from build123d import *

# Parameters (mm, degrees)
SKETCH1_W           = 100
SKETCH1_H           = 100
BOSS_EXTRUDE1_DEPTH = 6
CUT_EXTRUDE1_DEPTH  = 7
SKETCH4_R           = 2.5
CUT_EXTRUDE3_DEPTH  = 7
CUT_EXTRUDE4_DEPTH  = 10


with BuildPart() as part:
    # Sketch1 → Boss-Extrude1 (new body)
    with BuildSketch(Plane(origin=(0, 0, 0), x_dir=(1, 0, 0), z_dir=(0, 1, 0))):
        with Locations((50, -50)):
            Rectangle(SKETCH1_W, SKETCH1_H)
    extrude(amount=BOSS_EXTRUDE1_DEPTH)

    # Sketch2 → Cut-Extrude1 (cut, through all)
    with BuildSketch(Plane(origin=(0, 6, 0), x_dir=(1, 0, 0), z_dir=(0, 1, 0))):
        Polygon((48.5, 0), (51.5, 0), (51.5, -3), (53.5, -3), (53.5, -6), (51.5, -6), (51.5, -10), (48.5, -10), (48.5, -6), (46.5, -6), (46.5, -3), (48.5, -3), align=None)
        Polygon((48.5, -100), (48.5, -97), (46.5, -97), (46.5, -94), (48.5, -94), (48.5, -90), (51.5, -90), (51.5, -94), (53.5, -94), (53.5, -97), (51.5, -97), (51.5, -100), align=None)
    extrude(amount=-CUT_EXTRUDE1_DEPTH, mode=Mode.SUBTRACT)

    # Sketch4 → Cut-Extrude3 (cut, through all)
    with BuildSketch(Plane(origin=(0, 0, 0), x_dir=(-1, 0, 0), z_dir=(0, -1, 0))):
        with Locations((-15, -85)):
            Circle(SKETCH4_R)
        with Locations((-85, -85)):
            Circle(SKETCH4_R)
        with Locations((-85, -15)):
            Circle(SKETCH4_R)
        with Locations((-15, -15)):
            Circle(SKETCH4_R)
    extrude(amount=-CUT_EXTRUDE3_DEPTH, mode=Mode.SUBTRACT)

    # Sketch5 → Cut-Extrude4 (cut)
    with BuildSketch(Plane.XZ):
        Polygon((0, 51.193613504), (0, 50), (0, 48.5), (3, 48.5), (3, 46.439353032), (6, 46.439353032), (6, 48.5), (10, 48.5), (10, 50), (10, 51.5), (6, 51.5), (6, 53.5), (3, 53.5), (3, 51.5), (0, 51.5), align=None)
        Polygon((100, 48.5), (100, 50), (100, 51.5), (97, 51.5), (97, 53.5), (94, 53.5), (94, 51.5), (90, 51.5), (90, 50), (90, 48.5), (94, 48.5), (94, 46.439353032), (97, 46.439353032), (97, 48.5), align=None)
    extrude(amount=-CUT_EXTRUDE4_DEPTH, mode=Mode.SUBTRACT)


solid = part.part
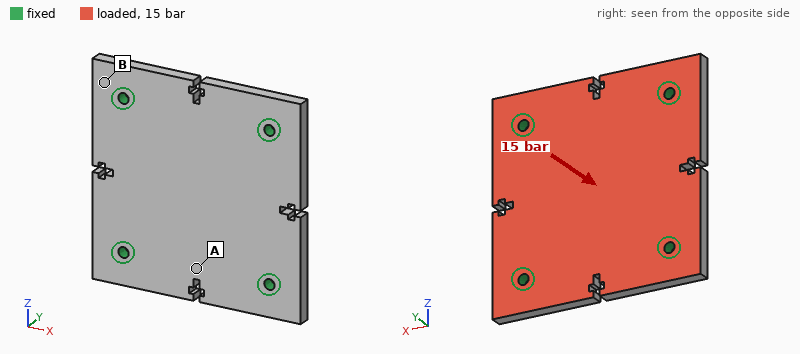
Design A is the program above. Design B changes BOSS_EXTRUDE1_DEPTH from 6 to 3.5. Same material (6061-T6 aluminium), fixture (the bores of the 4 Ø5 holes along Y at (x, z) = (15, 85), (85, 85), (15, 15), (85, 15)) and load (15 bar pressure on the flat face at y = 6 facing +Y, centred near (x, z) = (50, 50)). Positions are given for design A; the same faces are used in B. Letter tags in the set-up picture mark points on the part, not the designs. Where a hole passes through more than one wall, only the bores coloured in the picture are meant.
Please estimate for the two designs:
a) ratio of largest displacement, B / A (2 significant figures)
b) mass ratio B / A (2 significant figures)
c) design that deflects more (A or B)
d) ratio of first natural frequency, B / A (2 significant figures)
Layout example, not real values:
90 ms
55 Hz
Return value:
4.5
0.58
B
0.62
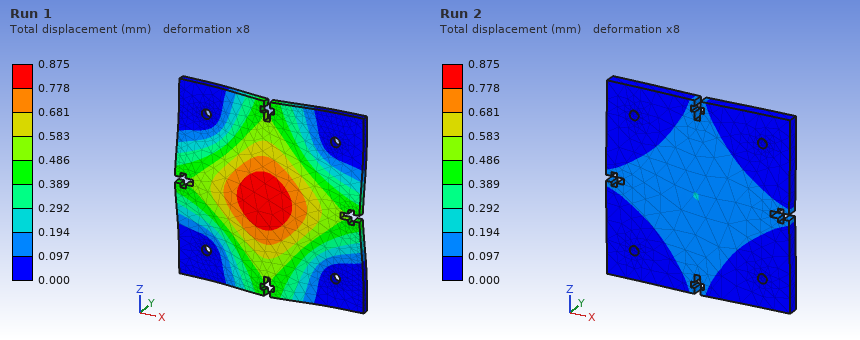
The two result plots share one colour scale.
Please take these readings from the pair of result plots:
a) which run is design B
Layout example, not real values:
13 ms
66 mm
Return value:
Run 1
